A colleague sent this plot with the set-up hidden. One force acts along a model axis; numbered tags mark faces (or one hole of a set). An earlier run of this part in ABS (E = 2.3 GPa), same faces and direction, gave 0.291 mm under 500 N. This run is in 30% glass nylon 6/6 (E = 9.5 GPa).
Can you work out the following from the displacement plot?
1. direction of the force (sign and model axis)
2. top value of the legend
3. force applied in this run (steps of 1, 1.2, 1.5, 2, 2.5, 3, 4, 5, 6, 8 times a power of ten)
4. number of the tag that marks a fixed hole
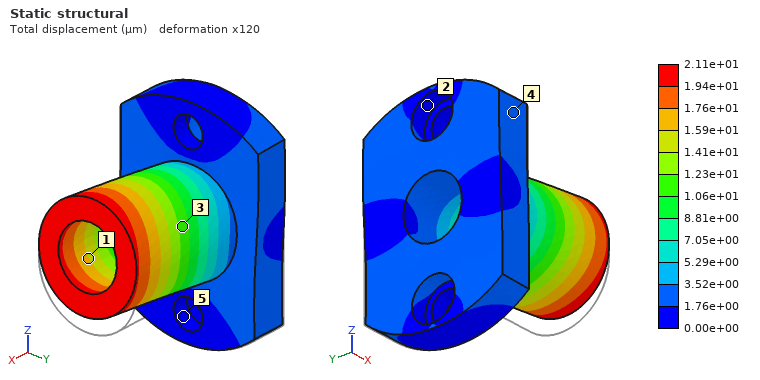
+Z
2.11e+01 µm
150 N
5
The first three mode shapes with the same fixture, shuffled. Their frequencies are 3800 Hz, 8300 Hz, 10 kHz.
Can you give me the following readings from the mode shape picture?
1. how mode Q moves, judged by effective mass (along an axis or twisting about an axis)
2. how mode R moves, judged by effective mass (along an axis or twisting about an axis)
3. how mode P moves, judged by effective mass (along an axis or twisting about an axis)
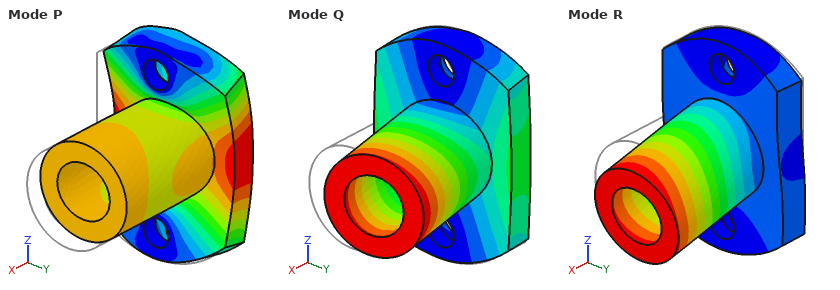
along Y
along Z
along X
